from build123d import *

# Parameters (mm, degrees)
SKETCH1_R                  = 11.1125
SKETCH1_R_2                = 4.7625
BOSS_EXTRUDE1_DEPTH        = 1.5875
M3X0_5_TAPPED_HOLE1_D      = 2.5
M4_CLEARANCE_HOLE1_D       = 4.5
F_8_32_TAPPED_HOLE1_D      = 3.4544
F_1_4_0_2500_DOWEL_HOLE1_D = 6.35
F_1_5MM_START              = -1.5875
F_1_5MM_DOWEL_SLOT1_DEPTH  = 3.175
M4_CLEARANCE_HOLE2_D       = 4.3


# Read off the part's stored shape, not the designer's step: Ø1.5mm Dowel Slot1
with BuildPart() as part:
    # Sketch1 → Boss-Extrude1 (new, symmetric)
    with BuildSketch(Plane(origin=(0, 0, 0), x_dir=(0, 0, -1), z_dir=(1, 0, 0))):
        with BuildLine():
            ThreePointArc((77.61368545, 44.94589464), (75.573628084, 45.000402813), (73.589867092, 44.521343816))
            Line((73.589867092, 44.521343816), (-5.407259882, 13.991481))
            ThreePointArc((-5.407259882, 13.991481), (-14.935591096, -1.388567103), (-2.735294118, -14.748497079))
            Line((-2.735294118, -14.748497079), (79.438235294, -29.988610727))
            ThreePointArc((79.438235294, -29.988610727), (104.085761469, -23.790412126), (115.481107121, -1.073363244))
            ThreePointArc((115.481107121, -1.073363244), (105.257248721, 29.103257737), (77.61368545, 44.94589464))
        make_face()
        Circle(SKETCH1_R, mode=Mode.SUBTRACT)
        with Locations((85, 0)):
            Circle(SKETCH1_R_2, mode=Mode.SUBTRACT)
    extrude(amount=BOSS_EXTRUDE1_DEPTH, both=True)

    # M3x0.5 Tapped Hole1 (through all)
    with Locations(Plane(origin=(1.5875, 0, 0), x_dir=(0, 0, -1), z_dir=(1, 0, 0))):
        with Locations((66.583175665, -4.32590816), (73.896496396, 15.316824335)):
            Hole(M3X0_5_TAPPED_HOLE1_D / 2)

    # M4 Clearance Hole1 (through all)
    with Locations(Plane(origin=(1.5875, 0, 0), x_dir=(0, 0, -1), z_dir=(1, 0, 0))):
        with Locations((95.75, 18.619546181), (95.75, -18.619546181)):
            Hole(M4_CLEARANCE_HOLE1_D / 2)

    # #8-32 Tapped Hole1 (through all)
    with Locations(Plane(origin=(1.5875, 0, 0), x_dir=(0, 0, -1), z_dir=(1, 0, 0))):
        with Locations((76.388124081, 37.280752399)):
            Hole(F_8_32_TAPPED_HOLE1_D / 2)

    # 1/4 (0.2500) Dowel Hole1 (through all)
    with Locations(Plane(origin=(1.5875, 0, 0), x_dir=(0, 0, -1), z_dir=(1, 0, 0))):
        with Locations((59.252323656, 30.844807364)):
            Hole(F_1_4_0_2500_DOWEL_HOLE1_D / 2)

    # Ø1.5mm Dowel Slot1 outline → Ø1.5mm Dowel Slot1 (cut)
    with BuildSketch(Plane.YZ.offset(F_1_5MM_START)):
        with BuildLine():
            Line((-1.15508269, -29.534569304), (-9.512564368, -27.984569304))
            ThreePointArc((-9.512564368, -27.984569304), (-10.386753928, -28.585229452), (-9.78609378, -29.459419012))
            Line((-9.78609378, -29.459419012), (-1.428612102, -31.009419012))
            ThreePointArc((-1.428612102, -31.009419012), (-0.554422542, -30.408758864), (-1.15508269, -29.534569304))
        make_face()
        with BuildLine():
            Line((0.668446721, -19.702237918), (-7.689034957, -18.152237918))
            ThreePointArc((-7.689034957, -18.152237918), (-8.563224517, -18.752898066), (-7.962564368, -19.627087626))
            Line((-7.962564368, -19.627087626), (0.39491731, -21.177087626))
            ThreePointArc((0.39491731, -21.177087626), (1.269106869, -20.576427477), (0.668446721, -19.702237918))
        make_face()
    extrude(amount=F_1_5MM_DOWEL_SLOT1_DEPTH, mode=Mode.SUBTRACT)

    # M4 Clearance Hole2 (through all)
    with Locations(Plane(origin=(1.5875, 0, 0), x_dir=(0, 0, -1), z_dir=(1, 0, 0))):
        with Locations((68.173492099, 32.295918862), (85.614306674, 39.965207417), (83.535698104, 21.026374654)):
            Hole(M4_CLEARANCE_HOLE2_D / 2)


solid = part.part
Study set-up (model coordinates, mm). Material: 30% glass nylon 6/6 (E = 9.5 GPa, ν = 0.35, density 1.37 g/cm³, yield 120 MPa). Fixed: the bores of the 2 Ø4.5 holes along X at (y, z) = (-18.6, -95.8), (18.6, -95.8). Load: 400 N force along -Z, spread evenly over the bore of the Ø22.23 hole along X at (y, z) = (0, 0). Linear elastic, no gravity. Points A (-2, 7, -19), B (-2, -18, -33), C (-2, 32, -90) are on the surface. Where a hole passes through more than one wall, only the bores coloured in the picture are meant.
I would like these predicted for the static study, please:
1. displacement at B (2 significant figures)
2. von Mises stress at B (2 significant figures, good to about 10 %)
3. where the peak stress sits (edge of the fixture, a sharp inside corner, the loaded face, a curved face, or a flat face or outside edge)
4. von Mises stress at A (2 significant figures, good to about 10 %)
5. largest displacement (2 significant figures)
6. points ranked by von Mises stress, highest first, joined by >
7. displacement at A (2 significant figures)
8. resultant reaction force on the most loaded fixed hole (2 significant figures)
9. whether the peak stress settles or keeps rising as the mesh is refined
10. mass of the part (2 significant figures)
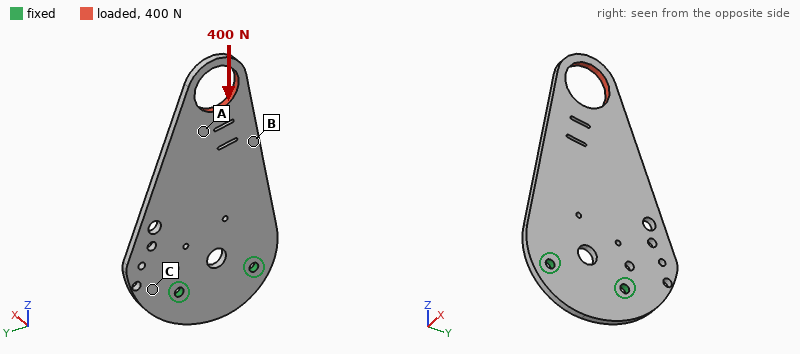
21 µm
4.5 MPa
a sharp inside corner
2.6 MPa
76 µm
B > A > C
21 µm
200 N
keeps rising
27 g
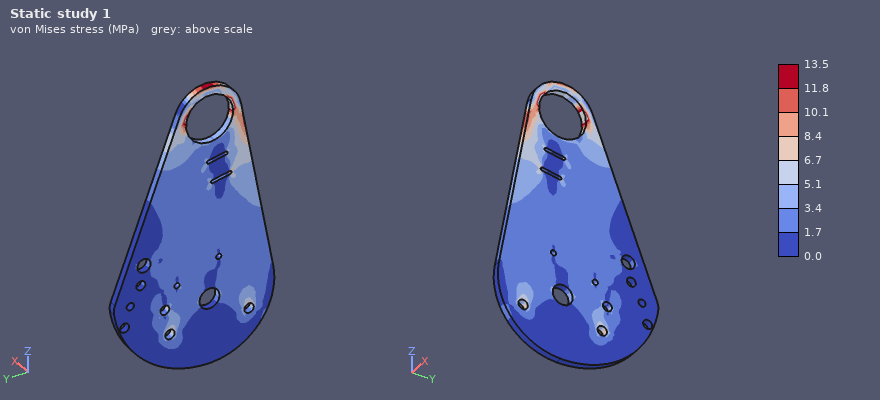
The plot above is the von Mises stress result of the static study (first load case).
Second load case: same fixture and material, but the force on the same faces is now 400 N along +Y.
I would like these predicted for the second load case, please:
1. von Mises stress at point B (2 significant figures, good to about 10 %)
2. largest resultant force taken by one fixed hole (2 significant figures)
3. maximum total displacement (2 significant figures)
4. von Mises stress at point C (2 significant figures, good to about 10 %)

11 MPa
990 N
0.60 mm
7.1 MPa
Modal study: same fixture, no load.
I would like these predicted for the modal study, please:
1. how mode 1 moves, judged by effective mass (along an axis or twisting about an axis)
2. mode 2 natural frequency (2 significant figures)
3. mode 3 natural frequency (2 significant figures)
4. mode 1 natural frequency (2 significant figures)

along X
690 Hz
840 Hz
170 Hz
